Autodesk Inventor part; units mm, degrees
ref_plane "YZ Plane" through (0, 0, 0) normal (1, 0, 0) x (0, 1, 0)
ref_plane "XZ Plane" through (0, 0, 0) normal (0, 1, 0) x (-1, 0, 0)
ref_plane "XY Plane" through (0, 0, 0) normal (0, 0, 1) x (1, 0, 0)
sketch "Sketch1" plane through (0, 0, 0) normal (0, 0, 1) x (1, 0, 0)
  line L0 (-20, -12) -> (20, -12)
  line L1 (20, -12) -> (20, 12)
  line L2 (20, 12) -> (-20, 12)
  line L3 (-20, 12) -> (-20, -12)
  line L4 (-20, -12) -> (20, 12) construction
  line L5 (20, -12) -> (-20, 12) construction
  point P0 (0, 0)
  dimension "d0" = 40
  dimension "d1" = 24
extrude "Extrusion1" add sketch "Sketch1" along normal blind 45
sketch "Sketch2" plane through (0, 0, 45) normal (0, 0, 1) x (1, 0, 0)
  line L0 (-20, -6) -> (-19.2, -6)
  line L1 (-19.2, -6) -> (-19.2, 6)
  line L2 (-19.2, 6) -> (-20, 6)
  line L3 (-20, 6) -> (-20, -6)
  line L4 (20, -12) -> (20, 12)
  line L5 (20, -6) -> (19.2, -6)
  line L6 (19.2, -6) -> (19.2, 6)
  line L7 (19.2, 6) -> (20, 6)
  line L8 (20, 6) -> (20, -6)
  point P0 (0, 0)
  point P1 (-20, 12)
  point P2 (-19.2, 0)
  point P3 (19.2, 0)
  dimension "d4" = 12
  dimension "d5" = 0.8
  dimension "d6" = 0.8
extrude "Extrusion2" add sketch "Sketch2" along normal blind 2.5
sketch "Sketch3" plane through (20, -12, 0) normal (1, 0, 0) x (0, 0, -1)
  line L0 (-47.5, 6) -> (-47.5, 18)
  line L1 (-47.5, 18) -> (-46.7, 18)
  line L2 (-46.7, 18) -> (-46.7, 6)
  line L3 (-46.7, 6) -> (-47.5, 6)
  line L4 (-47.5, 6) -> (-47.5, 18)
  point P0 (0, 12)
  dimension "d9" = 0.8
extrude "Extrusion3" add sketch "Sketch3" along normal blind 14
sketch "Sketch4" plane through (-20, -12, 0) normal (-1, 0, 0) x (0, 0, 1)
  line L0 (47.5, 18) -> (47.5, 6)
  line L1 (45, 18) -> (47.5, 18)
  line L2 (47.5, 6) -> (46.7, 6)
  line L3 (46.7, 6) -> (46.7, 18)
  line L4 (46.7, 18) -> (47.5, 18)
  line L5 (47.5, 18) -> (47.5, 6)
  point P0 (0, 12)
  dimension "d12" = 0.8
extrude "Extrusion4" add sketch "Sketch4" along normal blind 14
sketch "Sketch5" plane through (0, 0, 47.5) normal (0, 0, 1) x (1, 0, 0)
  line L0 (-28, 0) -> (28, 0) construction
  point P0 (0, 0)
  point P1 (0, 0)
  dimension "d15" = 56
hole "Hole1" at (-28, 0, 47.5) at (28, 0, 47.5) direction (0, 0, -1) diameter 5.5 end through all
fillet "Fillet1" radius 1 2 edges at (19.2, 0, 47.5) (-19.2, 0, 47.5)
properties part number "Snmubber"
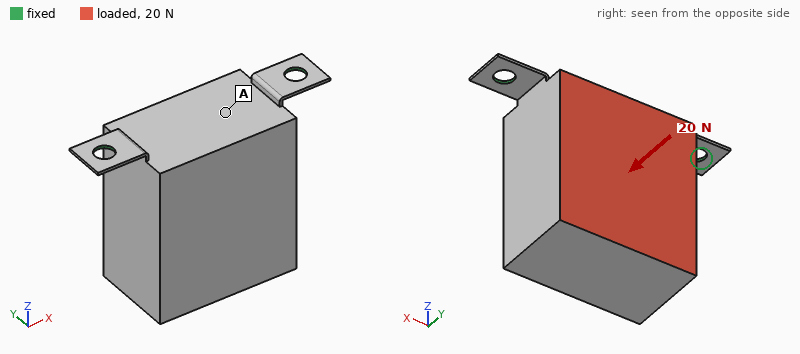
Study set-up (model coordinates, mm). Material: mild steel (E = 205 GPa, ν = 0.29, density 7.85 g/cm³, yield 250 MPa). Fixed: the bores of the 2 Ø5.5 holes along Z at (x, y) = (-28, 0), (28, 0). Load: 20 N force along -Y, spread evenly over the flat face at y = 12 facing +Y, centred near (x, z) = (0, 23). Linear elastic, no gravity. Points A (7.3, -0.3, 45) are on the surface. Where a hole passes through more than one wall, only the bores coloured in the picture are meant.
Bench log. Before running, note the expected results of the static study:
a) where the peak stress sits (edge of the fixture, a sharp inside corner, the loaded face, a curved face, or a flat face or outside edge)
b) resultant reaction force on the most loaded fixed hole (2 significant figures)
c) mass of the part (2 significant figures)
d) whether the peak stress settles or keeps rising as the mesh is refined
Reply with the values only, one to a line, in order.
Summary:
edge of the fixture
10 N
340 g
keeps rising
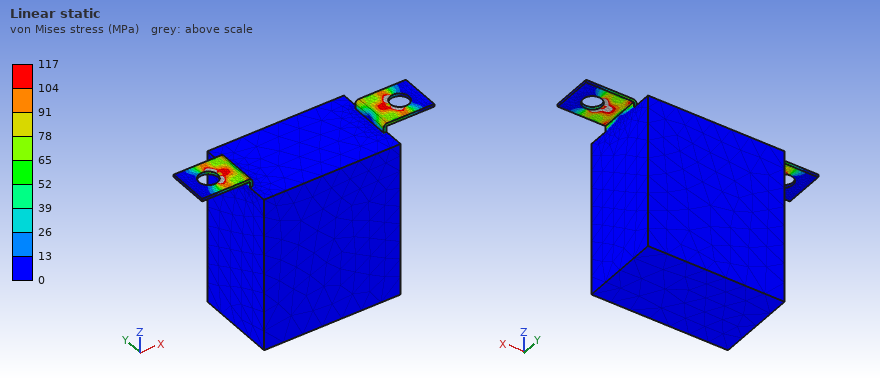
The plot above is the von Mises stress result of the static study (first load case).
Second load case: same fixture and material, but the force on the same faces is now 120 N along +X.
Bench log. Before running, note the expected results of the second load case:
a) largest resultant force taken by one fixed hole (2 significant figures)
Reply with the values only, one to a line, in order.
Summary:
95 N
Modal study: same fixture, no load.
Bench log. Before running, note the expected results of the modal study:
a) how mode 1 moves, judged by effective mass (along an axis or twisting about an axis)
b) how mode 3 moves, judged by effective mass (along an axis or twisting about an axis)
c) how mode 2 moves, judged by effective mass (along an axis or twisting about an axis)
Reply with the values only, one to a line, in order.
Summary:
along Y
along Z
along X
